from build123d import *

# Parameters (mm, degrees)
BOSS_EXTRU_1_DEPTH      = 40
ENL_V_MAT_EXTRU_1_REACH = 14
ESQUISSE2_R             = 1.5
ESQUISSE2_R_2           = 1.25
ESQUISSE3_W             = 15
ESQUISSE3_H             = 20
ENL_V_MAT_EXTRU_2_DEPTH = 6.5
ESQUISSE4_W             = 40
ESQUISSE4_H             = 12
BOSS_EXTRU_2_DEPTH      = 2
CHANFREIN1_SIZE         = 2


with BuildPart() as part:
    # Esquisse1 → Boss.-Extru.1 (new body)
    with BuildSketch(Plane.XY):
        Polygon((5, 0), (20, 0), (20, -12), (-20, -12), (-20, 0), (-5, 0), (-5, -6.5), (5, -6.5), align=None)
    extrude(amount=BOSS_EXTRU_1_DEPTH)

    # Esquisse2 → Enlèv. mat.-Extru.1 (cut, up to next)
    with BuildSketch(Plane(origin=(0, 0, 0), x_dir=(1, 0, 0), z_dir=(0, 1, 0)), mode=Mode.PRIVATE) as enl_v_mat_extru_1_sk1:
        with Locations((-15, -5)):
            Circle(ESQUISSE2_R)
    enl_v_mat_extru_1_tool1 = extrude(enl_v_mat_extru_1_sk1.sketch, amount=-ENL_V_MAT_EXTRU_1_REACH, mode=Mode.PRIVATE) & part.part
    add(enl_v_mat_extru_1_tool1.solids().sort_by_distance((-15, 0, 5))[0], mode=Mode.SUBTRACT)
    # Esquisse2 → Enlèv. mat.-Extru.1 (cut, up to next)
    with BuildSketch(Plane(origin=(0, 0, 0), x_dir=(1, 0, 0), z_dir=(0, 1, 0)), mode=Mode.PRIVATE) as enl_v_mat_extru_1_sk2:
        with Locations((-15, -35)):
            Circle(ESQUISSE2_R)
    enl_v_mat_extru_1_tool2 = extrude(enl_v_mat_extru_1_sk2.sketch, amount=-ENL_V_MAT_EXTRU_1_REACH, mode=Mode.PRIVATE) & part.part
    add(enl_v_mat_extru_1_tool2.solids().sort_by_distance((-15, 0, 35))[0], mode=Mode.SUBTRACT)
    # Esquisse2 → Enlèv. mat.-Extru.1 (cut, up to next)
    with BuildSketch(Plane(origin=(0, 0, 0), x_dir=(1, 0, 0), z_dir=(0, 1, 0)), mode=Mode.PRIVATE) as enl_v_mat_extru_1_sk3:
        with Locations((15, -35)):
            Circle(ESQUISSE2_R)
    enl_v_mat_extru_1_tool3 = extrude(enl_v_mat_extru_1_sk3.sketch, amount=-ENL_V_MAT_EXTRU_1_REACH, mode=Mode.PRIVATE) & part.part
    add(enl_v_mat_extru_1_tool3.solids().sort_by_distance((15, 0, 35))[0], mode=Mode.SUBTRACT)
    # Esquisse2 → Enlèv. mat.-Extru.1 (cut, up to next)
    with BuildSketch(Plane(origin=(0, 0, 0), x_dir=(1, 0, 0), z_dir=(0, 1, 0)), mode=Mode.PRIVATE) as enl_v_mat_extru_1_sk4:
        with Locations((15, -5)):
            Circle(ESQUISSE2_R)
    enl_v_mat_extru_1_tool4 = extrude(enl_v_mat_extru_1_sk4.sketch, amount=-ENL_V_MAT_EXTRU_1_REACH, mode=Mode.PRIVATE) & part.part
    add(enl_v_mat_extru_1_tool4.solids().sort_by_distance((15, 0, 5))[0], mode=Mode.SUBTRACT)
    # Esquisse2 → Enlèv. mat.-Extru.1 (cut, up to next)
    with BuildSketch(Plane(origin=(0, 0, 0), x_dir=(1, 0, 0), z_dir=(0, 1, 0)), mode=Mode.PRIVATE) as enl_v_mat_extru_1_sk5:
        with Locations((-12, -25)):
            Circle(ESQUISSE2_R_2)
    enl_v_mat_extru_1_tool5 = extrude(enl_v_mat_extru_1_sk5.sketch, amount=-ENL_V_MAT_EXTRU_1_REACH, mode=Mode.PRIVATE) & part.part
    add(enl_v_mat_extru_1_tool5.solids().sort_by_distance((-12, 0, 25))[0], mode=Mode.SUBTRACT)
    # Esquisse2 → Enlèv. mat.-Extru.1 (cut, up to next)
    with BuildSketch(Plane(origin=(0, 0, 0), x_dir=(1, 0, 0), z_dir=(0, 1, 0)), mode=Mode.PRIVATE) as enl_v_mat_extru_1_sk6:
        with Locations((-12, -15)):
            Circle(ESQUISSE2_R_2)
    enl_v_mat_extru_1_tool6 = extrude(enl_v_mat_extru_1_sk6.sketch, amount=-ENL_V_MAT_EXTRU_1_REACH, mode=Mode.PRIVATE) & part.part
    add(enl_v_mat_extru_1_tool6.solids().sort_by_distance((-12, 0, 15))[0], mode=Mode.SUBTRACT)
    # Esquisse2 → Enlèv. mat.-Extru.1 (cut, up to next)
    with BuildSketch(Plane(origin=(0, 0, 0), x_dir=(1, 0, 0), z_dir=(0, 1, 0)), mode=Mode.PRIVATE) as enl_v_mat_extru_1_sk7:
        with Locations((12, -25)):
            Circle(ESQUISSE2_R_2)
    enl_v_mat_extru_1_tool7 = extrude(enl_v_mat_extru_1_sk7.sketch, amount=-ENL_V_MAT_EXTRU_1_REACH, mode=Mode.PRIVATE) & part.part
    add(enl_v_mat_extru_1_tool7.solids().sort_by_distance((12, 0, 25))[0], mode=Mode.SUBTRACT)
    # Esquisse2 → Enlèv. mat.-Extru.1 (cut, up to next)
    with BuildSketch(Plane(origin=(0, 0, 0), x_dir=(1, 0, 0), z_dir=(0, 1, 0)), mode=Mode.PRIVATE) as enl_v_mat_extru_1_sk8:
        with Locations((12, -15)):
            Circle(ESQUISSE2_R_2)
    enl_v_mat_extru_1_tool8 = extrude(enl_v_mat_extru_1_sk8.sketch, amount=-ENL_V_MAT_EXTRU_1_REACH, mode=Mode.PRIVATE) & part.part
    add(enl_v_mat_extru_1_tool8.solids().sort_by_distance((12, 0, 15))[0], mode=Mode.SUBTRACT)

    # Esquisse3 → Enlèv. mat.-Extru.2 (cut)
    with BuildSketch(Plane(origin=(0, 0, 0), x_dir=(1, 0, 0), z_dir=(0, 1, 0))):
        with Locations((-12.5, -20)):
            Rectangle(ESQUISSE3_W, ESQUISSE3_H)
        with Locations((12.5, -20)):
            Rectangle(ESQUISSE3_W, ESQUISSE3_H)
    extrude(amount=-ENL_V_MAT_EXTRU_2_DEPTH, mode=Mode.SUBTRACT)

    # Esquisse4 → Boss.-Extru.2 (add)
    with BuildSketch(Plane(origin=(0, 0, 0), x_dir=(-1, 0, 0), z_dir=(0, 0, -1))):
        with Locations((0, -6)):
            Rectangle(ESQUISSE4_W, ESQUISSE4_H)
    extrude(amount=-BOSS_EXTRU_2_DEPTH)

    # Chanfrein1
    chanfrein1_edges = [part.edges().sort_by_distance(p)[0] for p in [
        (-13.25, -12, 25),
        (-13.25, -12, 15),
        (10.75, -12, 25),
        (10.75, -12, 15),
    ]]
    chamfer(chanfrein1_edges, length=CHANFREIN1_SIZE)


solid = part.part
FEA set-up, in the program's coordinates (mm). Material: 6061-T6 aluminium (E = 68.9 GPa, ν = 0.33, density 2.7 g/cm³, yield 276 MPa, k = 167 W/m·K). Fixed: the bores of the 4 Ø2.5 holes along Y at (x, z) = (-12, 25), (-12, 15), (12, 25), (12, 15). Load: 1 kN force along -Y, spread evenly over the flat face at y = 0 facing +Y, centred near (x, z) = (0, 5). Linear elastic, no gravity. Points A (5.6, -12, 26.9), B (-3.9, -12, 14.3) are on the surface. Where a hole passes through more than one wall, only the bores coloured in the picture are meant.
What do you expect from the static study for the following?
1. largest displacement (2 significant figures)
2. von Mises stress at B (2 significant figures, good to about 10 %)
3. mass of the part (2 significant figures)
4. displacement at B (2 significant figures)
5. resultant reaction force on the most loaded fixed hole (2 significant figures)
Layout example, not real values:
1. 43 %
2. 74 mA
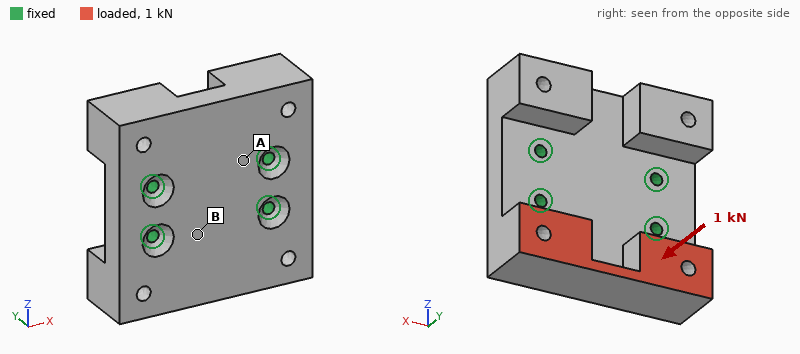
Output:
1. 39 µm
2. 30 MPa
3. 33 g
4. 5.8 µm
5. 790 N
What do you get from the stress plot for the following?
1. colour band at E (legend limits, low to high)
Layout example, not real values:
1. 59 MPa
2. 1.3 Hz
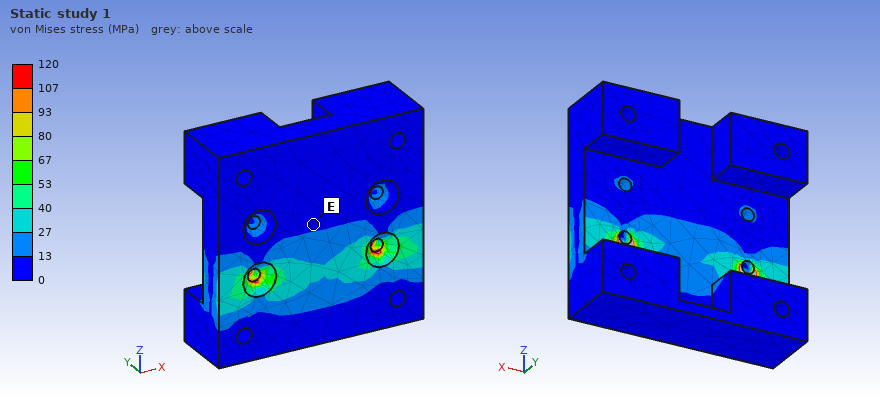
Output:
1. 0 to 13 MPa
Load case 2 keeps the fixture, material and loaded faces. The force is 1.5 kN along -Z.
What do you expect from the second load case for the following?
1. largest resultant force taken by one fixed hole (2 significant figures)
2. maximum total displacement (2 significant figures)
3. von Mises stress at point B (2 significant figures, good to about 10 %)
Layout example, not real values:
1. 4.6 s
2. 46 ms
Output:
1. 850 N
2. 66 µm
3. 47 MPa
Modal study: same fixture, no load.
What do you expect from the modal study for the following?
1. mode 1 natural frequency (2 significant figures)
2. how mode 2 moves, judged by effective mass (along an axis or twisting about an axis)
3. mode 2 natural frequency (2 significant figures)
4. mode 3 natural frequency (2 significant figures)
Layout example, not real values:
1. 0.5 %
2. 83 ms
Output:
1. 8800 Hz
2. along Y
3. 9400 Hz
4. 13 kHz
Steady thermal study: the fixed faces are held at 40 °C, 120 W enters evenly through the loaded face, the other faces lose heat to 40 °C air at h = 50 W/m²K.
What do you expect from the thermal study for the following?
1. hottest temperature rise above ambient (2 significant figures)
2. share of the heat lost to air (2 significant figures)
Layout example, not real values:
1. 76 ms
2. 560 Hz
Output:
1. 56 K
2. 4.0 %
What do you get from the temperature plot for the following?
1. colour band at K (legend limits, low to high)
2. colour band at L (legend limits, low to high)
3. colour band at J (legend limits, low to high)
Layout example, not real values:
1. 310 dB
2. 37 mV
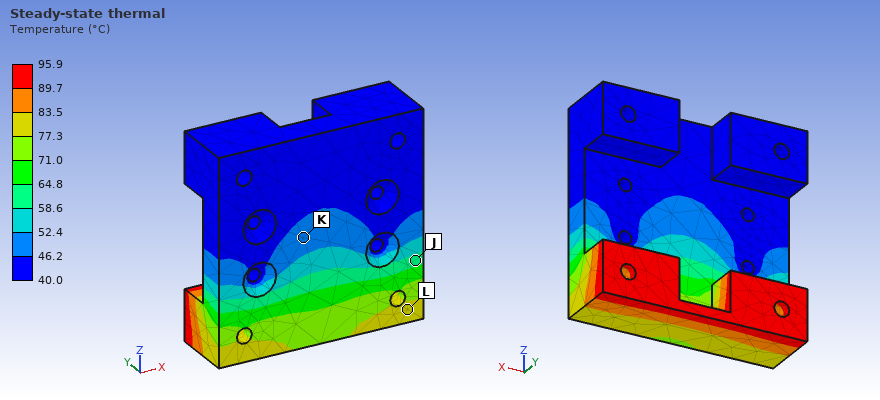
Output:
1. 46.2 to 52.4 °C
2. 77.3 to 83.5 °C
3. 58.6 to 64.8 °C
